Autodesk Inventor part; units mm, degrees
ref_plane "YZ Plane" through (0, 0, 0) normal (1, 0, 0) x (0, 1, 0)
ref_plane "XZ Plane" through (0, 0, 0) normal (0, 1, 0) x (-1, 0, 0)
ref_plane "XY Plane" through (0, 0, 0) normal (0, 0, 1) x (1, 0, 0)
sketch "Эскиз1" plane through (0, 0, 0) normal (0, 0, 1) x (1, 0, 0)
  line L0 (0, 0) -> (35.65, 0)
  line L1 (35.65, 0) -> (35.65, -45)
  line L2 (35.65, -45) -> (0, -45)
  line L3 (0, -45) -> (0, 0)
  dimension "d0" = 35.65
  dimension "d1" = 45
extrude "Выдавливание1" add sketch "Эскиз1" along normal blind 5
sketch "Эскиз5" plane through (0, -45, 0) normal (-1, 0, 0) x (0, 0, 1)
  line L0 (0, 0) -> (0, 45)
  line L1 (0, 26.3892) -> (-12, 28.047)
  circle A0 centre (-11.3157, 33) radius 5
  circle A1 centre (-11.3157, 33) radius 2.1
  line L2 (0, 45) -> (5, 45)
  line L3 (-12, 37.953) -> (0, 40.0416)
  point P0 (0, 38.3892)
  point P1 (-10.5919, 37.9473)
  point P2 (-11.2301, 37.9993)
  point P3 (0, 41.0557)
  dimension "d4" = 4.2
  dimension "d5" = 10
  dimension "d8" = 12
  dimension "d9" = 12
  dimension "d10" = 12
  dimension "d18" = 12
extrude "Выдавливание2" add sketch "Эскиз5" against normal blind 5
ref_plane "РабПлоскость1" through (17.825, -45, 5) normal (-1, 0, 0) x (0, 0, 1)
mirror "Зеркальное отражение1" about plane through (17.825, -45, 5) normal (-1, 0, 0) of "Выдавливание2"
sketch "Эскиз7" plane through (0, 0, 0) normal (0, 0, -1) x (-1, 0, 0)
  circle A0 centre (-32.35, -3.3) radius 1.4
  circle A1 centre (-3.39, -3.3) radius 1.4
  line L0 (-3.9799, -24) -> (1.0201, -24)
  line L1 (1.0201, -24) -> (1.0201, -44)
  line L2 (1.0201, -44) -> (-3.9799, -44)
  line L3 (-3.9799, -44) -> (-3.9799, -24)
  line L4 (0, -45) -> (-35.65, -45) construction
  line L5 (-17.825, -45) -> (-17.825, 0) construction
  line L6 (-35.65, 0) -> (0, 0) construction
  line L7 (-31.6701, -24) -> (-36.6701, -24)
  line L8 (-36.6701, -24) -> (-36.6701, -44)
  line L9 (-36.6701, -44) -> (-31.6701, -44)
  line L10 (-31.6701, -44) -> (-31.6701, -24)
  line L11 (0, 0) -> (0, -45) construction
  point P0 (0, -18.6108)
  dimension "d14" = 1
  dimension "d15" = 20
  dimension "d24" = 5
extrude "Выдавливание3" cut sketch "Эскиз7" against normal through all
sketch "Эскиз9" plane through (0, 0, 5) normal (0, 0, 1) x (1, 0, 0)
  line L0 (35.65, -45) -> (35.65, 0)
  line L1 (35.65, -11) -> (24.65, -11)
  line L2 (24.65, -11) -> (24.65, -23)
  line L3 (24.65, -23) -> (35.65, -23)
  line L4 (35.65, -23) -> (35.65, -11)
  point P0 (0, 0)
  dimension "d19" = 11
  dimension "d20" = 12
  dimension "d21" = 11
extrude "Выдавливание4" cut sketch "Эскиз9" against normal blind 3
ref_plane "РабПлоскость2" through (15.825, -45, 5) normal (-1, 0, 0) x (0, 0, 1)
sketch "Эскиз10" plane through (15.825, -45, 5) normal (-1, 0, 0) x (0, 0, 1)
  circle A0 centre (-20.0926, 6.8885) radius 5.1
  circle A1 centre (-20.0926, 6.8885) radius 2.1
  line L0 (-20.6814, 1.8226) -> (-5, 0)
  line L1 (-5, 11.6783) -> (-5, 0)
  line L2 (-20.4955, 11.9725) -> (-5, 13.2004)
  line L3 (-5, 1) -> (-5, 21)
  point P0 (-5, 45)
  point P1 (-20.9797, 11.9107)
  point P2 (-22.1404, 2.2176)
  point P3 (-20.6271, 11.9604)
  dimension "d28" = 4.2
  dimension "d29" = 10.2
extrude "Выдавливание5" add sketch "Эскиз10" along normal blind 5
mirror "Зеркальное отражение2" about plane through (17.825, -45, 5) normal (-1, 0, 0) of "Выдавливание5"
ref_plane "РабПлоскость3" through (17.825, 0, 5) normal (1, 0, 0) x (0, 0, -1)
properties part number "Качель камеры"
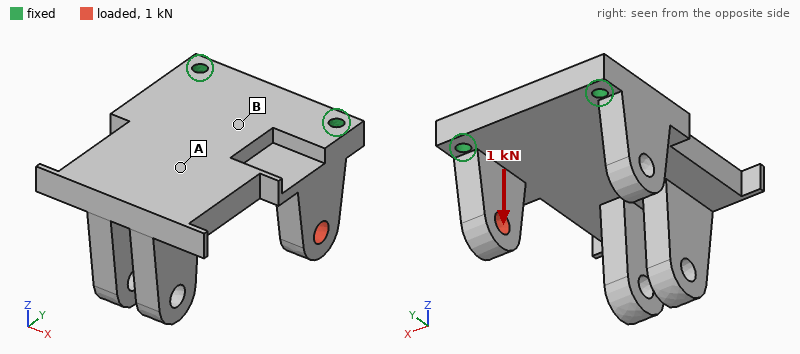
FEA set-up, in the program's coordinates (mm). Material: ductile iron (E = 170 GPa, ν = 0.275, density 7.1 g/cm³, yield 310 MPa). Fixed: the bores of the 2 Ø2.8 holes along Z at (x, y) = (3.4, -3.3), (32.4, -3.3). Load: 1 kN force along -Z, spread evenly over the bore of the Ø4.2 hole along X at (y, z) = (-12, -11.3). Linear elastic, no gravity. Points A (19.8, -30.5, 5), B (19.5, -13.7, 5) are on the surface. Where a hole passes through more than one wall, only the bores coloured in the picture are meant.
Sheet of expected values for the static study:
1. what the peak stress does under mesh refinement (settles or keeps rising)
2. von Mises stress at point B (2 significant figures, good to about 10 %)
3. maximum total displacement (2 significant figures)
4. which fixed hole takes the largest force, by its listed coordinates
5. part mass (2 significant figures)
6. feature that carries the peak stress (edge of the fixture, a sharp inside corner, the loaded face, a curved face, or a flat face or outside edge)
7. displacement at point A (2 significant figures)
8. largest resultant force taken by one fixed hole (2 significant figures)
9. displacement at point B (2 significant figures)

keeps rising
23 MPa
43 µm
(32.4, -3.3)
74 g
edge of the fixture
22 µm
1.0 kN
8.6 µm
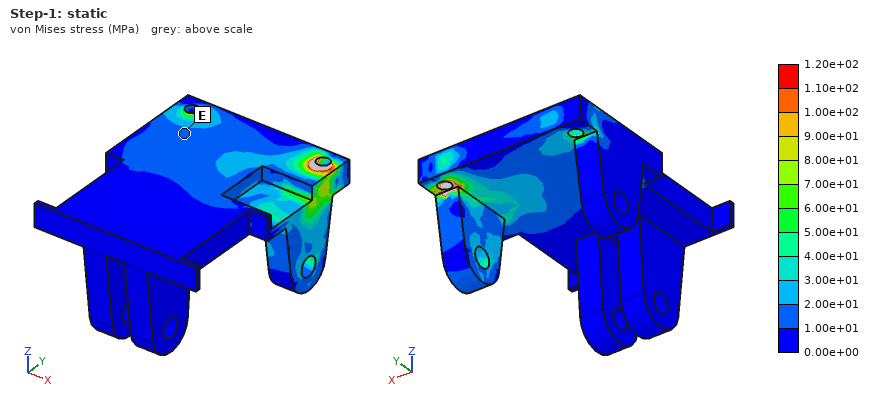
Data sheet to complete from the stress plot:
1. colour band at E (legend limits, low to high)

1.00e+01 to 2.00e+01 MPa
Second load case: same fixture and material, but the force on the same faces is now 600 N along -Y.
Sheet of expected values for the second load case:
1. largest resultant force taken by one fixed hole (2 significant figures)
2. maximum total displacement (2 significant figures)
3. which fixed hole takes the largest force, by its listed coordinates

620 N
53 µm
(32.4, -3.3)
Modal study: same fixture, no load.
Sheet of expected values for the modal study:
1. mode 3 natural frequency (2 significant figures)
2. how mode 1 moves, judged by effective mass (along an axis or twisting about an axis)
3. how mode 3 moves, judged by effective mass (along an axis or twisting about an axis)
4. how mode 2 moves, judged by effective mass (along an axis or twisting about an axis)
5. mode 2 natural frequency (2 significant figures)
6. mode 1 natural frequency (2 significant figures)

6600 Hz
along Z
along Z
along X
4100 Hz
1600 Hz
